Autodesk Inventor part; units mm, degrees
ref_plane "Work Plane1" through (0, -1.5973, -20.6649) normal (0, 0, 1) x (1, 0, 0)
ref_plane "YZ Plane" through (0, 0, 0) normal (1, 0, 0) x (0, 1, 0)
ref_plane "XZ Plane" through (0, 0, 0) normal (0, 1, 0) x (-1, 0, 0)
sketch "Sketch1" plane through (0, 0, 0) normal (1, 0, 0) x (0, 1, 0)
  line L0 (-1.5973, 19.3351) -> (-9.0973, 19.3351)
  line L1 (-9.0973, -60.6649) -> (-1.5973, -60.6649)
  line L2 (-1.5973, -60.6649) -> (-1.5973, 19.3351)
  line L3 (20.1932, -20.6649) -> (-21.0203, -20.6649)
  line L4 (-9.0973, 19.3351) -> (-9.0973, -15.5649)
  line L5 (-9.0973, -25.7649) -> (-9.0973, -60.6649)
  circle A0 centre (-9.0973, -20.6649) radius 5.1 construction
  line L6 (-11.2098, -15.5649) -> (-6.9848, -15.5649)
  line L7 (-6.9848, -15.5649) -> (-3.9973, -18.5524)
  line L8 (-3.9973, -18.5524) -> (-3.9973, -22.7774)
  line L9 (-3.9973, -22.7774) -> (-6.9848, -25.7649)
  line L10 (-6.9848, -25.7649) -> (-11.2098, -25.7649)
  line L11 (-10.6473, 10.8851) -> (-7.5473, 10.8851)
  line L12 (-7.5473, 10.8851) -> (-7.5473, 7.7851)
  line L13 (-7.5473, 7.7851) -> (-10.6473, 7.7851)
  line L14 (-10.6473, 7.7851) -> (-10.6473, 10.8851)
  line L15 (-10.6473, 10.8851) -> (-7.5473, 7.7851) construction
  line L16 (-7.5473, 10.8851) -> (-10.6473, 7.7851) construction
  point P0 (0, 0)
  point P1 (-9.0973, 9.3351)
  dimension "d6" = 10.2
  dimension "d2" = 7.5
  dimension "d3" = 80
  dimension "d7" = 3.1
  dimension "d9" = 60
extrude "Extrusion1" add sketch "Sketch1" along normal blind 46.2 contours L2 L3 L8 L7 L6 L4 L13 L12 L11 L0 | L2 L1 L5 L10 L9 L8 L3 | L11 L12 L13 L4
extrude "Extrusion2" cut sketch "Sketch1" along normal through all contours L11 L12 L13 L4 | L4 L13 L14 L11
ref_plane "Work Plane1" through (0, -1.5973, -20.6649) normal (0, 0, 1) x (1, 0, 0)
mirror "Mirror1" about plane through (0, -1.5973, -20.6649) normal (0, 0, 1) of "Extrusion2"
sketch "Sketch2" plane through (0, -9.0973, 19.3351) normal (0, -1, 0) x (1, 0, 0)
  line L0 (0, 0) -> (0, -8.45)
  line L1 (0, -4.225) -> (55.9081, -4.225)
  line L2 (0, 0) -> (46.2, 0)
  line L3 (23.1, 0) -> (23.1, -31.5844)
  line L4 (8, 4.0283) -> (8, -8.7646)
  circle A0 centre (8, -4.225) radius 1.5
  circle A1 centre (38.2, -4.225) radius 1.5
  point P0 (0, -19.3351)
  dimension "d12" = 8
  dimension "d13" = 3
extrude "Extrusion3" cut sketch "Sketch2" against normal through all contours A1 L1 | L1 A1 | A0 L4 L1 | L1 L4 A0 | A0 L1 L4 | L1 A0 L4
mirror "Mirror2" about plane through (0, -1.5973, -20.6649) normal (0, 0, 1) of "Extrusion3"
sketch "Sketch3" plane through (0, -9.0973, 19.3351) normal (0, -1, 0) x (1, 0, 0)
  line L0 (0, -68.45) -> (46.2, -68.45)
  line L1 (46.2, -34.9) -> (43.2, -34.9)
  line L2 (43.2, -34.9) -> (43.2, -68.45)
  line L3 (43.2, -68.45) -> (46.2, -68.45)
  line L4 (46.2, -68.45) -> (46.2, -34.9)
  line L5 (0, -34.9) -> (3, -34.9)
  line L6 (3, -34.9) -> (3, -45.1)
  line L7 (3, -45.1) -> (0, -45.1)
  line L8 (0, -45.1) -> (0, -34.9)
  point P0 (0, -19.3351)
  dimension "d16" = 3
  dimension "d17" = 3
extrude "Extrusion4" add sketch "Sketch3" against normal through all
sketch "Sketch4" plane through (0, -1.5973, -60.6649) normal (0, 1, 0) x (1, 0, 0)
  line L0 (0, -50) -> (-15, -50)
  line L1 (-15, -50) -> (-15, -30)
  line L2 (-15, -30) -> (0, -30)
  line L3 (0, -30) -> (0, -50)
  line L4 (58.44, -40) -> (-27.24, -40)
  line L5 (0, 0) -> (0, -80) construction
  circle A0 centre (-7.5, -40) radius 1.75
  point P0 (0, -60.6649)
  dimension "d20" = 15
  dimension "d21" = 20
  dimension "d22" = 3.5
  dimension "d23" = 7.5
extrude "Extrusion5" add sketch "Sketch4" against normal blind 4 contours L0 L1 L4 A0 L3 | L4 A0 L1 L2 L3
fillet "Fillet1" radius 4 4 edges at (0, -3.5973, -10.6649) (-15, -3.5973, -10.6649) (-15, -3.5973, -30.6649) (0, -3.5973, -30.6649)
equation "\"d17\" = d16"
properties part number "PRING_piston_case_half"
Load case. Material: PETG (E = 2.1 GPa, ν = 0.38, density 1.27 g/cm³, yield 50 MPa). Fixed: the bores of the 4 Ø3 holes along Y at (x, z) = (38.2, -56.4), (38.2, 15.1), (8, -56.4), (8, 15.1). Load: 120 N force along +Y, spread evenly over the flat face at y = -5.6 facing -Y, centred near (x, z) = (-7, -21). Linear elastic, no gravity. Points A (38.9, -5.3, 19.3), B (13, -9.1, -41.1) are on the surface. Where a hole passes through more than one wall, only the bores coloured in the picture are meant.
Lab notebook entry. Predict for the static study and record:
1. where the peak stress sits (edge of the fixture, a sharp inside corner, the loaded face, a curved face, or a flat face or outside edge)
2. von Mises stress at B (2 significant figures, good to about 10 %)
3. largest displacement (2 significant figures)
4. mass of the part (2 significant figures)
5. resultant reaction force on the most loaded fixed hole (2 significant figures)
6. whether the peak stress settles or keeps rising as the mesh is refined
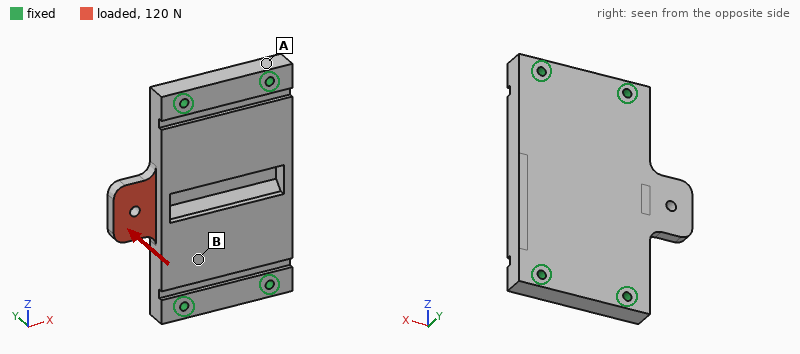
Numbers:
edge of the fixture
4.2 MPa
1.0 mm
34 g
92 N
keeps rising
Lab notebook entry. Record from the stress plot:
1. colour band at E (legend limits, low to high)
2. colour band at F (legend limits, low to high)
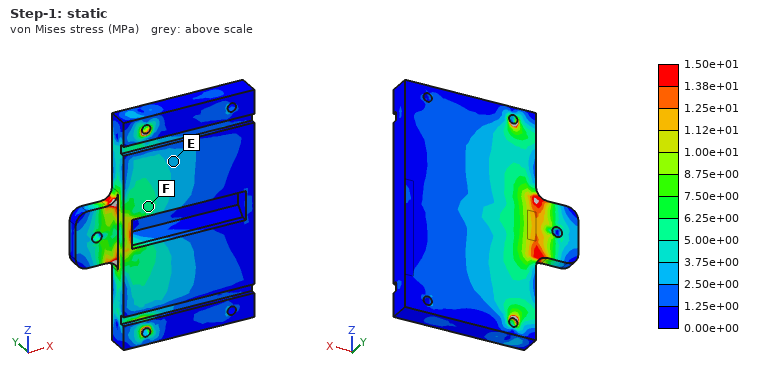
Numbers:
2.50e+00 to 3.75e+00 MPa
5.00e+00 to 6.25e+00 MPa
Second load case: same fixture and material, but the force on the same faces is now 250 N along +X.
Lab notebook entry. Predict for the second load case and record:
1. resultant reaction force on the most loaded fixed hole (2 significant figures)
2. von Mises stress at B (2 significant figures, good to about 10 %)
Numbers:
90 N
0.98 MPa
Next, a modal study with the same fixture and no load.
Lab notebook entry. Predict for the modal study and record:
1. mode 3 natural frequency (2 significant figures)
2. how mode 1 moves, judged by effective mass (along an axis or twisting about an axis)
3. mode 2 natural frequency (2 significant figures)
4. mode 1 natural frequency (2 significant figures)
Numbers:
3200 Hz
along Y
1700 Hz
1200 Hz
